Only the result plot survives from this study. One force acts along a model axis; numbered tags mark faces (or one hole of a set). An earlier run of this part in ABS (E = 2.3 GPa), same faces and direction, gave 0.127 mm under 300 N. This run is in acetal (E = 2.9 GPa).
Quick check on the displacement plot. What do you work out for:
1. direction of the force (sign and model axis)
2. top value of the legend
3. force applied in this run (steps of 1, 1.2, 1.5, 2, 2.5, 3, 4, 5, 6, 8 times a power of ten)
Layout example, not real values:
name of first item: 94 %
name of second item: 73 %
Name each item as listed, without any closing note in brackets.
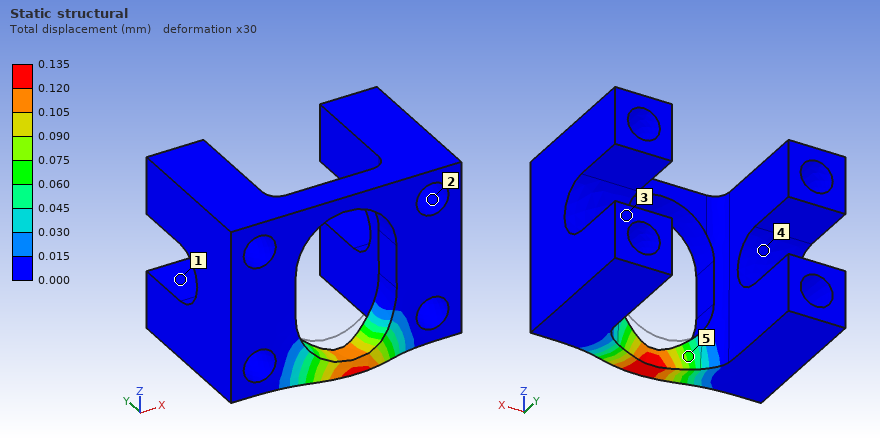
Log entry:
direction of the force: -Y
top value of the legend: 0.135 mm
force applied in this run: 400 N
